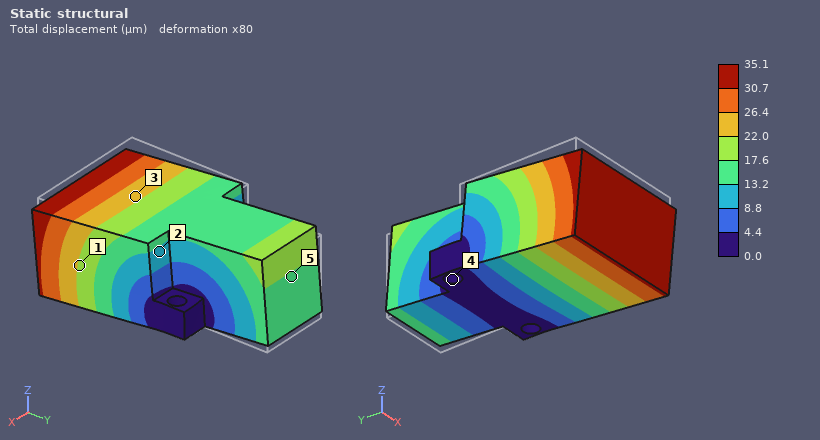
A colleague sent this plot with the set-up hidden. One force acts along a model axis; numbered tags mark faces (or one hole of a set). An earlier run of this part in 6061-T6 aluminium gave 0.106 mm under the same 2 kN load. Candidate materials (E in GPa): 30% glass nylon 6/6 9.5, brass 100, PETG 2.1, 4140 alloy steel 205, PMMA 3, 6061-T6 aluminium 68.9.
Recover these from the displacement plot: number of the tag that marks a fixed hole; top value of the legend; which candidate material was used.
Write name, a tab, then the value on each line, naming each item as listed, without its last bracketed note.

number of the tag that marks a fixed hole	4
top value of the legend	35.1 µm
which candidate material was used	4140 alloy steel
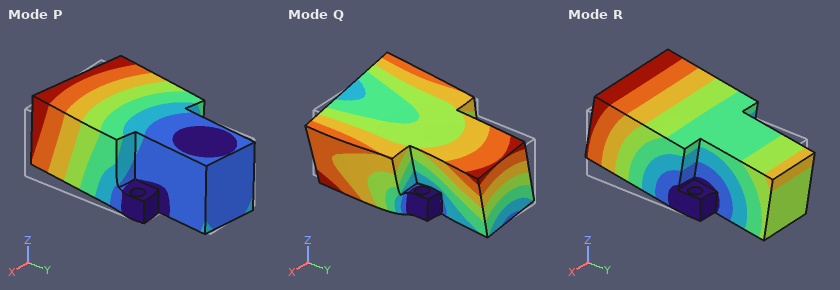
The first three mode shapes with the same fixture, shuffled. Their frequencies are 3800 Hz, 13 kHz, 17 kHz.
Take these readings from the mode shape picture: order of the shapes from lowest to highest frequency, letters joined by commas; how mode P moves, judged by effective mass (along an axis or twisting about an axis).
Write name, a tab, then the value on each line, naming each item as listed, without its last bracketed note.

order of the shapes from lowest to highest frequency, letters joined by commas	R, P, Q
how mode P moves, judged by effective mass	along X
